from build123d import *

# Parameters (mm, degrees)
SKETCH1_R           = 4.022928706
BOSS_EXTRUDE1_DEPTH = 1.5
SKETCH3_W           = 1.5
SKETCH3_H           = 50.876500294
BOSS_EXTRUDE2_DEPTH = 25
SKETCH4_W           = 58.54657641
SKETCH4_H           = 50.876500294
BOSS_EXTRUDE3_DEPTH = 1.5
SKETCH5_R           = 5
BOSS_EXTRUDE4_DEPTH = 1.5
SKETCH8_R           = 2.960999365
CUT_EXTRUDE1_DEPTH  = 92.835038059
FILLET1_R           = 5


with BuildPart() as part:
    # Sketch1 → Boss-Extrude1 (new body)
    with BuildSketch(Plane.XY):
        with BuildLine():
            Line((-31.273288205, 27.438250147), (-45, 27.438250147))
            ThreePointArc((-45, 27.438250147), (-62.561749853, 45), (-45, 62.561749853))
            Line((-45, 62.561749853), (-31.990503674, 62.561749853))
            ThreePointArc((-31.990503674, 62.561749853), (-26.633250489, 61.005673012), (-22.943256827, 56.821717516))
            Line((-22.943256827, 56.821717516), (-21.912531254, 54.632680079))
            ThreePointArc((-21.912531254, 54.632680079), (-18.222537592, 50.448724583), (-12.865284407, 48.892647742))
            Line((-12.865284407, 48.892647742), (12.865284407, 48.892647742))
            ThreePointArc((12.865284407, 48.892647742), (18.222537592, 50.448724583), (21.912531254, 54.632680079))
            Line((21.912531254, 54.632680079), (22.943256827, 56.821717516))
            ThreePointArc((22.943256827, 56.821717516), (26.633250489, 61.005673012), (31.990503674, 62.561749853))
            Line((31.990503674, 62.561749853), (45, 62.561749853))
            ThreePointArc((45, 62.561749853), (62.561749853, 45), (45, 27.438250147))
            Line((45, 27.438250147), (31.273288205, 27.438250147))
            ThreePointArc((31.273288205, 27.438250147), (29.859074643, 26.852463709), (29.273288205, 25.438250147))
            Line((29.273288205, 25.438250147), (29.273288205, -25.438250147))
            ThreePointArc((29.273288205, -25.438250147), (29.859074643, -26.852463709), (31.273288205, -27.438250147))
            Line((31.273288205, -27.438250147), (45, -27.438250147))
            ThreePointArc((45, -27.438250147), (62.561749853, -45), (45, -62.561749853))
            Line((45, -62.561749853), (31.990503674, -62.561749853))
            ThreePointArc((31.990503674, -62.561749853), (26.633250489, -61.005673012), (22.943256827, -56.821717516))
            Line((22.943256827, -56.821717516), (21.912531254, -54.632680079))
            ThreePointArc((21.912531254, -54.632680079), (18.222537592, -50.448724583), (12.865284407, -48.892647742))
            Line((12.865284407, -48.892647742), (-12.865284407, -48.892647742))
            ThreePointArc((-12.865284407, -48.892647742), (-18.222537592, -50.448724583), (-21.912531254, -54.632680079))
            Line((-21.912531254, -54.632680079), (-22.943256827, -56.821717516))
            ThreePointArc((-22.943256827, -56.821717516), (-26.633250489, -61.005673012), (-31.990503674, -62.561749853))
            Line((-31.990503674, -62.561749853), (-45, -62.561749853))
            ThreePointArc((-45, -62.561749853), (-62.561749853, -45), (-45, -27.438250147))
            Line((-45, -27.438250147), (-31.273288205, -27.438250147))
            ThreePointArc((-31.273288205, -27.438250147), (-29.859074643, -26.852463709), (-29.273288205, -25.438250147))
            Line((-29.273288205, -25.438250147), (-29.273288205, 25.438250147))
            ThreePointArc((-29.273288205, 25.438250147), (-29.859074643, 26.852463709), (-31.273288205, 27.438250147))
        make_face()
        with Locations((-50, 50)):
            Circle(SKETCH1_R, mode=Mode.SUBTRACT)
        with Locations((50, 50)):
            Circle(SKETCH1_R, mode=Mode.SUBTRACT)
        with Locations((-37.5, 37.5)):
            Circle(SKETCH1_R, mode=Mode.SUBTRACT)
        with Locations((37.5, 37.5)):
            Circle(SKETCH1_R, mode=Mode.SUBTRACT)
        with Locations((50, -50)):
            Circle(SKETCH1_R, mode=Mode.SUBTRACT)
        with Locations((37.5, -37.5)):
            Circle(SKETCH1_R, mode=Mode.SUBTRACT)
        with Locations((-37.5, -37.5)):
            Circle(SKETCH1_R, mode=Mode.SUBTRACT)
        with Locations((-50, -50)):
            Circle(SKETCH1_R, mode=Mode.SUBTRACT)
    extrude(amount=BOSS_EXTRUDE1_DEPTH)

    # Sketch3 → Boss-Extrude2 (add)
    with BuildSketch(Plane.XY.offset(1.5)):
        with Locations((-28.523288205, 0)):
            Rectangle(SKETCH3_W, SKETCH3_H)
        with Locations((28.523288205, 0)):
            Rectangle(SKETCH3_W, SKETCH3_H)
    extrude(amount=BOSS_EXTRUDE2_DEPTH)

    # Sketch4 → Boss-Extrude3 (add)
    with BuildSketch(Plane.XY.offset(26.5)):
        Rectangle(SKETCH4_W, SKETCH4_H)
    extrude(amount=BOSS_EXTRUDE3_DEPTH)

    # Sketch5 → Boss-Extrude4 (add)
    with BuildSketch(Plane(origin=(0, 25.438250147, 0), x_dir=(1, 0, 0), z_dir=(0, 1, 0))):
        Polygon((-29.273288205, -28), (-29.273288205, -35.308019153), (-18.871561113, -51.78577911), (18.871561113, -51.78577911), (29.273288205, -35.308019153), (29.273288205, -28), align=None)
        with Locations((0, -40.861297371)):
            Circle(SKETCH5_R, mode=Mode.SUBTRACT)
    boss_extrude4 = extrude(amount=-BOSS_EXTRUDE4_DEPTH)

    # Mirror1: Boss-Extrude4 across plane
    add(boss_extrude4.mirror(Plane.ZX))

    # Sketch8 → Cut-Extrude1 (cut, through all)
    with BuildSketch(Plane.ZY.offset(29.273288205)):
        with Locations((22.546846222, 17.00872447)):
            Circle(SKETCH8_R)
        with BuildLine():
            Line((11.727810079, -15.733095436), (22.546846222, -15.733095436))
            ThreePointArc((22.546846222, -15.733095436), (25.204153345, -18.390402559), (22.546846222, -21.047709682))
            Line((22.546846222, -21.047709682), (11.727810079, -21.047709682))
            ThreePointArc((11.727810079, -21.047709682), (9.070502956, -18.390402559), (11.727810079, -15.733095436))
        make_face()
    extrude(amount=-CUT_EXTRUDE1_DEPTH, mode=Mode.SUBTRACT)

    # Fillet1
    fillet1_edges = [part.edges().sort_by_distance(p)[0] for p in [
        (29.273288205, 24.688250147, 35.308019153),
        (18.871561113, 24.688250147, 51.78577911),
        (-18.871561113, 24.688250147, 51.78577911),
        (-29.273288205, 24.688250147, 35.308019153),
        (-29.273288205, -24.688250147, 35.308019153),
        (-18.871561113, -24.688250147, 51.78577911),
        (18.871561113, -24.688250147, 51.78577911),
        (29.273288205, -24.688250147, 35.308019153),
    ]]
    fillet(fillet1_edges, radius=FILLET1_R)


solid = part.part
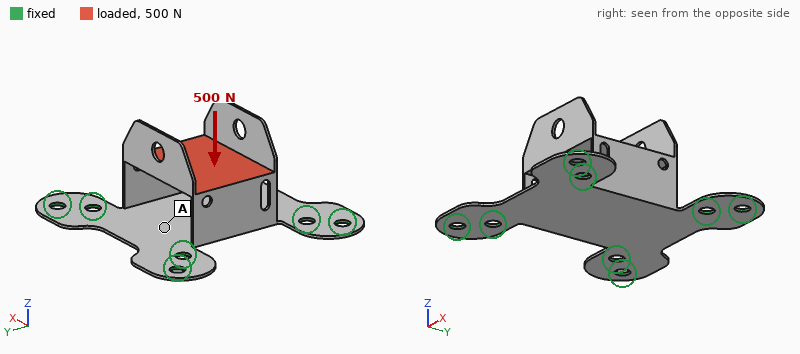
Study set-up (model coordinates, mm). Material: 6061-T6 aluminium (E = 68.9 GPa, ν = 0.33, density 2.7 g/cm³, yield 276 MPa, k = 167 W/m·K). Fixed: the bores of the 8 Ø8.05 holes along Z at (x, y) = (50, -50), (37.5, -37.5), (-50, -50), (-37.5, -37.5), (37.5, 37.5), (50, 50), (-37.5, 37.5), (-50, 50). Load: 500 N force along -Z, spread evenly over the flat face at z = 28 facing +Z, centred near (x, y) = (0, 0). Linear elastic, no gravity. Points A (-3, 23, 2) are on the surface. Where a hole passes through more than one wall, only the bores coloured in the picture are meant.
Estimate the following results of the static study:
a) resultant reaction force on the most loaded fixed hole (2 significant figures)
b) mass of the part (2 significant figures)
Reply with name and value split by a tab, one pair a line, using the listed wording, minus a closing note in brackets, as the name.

resultant reaction force on the most loaded fixed hole	140 N
mass of the part	71 g
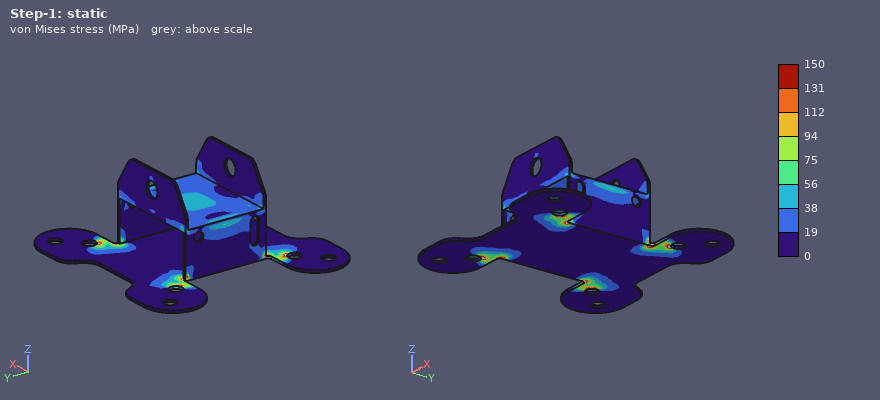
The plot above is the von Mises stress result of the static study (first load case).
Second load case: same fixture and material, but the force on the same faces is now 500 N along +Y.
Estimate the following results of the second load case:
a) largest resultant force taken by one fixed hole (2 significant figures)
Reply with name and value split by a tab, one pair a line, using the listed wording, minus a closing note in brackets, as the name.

largest resultant force taken by one fixed hole	180 N
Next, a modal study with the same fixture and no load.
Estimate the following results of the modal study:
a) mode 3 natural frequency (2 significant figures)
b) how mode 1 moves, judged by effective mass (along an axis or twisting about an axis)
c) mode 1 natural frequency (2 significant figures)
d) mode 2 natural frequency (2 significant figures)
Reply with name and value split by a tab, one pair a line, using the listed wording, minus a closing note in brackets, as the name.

mode 3 natural frequency	1300 Hz
how mode 1 moves, judged by effective mass	along X
mode 1 natural frequency	740 Hz
mode 2 natural frequency	1300 Hz
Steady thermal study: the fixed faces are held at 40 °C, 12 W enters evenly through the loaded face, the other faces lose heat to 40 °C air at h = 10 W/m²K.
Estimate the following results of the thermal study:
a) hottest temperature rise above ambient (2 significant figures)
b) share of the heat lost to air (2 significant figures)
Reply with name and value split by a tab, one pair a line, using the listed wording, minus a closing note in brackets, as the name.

hottest temperature rise above ambient	27 K
share of the heat lost to air	30 %
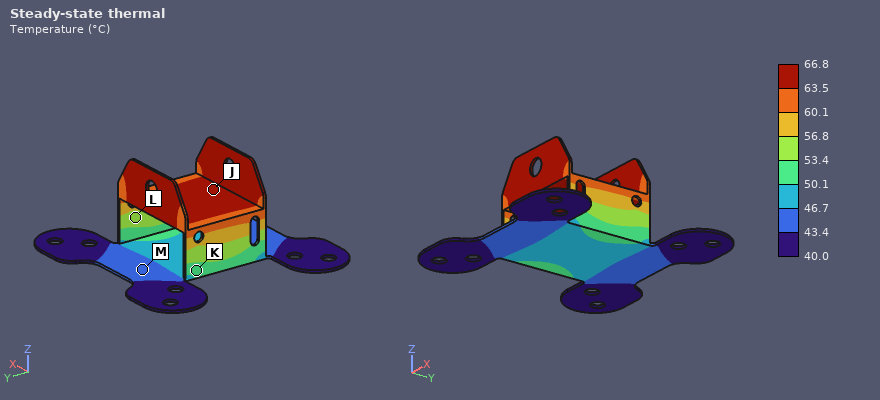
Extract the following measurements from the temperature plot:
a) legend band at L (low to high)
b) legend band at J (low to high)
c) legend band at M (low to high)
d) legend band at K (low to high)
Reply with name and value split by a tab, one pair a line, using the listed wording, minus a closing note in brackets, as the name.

legend band at L	53.4 to 56.8 °C
legend band at J	63.5 to 66.8 °C
legend band at M	43.4 to 46.7 °C
legend band at K	50.1 to 53.4 °C
